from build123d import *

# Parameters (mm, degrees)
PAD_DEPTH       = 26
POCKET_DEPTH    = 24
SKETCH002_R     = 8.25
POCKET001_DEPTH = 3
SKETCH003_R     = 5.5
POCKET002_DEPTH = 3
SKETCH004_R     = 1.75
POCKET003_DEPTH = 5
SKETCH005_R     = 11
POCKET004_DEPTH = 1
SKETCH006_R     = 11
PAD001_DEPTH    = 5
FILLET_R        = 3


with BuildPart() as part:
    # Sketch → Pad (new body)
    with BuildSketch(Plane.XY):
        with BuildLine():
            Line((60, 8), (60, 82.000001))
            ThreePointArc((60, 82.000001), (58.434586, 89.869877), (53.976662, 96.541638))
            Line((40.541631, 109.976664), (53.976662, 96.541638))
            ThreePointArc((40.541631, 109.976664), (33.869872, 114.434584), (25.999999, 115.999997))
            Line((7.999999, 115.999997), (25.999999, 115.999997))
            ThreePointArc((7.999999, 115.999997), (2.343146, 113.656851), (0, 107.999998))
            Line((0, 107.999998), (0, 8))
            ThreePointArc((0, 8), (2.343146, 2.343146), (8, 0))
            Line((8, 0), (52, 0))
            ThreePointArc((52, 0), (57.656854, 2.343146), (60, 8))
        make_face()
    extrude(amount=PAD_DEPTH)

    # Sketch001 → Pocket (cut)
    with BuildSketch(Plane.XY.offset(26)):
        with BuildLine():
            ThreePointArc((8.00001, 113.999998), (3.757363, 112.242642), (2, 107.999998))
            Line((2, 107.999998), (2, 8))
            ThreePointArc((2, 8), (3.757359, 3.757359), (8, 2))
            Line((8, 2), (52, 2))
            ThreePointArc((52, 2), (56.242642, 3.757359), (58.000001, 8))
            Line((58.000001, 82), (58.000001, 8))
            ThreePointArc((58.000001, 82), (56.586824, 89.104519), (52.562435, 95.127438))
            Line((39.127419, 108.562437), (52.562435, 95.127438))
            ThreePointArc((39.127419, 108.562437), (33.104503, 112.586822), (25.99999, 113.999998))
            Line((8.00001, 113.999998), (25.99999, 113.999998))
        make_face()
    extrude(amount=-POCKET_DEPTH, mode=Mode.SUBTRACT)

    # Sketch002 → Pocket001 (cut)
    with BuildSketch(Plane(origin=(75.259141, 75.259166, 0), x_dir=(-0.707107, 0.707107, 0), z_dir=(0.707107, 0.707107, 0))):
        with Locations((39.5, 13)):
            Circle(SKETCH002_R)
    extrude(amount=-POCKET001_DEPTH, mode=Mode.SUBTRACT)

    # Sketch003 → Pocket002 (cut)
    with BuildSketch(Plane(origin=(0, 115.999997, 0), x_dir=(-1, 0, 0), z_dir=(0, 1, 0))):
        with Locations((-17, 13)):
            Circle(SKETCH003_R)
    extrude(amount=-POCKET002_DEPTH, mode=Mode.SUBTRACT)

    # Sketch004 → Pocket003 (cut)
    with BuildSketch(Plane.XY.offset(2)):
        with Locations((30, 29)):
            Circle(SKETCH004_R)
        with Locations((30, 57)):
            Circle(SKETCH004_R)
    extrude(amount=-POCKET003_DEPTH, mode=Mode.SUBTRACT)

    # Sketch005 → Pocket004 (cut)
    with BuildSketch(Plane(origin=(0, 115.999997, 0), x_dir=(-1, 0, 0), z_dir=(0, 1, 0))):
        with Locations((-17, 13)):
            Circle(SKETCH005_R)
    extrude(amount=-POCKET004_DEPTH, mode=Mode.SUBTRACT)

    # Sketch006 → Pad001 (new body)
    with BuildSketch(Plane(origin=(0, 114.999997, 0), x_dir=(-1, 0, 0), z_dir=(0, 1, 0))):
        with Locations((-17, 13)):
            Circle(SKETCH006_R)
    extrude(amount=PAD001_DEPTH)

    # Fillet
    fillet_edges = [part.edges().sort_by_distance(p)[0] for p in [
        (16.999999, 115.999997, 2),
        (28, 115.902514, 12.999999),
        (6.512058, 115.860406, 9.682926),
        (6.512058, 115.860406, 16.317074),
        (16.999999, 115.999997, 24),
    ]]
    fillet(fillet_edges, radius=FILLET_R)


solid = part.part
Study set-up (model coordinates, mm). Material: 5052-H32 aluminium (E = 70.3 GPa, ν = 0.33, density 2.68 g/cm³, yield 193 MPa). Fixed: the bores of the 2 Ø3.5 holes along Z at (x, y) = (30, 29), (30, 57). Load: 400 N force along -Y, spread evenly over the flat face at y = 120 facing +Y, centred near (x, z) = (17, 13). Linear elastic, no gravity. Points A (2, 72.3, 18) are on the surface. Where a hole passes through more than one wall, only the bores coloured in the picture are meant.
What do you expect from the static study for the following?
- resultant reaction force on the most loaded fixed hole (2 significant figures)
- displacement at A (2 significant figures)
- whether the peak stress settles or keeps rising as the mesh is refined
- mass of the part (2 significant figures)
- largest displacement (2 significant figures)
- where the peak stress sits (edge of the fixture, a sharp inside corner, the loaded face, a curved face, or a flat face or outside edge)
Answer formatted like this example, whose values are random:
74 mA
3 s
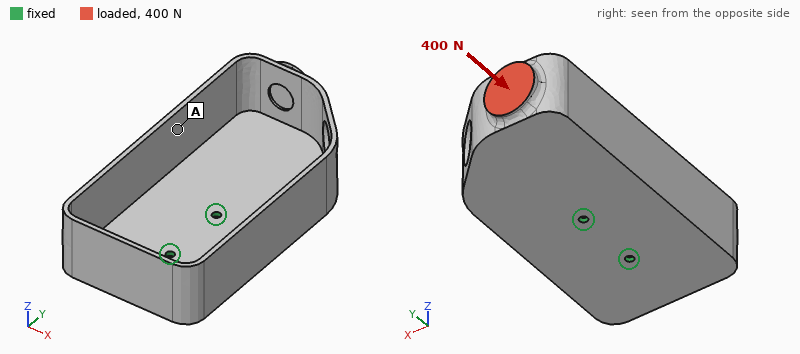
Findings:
310 N
0.15 mm
keeps rising
79 g
0.36 mm
edge of the fixture
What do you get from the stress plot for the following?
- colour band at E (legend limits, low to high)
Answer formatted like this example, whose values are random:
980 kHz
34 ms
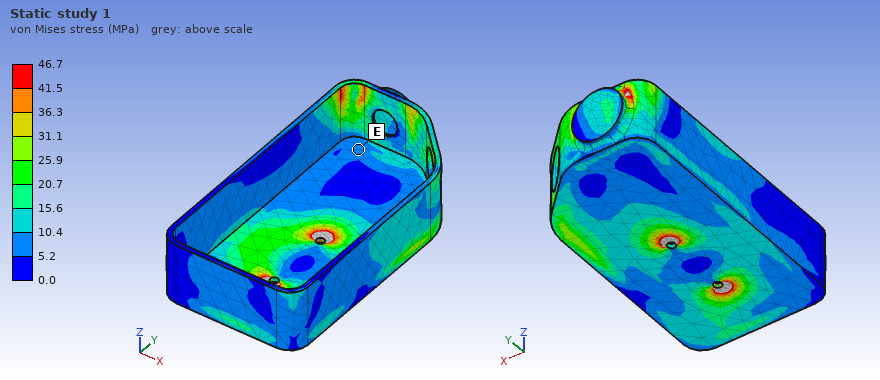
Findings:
5.2 to 10.4 MPa
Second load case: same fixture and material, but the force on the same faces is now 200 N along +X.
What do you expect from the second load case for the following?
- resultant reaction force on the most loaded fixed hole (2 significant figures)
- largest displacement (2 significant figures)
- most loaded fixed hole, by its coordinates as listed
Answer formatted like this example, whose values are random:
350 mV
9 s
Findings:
620 N
0.35 mm
(30, 57)
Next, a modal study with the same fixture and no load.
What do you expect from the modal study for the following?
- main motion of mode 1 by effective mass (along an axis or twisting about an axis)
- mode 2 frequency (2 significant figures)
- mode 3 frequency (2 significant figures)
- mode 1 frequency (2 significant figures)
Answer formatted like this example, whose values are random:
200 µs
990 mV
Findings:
along Z
560 Hz
950 Hz
450 Hz
